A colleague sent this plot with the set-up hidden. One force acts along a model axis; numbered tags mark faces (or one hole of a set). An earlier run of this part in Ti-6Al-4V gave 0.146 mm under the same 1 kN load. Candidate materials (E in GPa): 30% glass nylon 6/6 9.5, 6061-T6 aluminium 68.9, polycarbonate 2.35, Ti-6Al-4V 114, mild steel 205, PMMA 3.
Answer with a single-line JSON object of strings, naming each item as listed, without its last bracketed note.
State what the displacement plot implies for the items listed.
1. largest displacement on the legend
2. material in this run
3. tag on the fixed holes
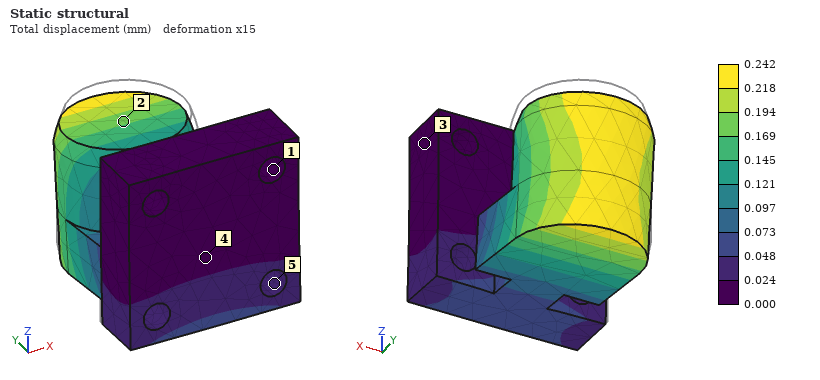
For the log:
{"largest displacement on the legend": "0.242 mm", "material in this run": "6061-T6 aluminium", "tag on the fixed holes": "1"}
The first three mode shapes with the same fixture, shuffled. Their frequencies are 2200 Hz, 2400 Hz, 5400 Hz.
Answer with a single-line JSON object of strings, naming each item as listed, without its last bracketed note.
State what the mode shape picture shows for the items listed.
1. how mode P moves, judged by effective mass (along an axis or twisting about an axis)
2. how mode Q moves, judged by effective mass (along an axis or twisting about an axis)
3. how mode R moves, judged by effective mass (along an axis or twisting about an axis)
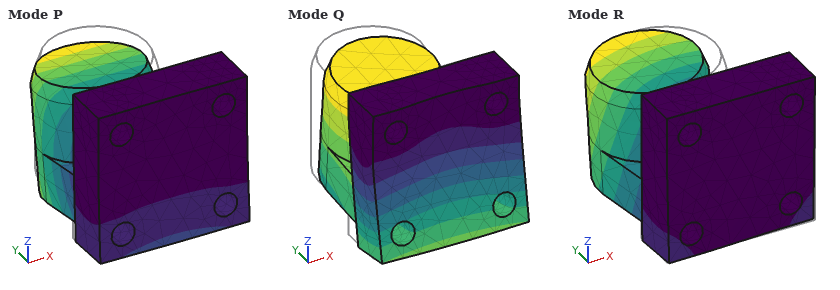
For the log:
{"how mode P moves, judged by effective mass": "along Z", "how mode Q moves, judged by effective mass": "along Y", "how mode R moves, judged by effective mass": "along X"}
